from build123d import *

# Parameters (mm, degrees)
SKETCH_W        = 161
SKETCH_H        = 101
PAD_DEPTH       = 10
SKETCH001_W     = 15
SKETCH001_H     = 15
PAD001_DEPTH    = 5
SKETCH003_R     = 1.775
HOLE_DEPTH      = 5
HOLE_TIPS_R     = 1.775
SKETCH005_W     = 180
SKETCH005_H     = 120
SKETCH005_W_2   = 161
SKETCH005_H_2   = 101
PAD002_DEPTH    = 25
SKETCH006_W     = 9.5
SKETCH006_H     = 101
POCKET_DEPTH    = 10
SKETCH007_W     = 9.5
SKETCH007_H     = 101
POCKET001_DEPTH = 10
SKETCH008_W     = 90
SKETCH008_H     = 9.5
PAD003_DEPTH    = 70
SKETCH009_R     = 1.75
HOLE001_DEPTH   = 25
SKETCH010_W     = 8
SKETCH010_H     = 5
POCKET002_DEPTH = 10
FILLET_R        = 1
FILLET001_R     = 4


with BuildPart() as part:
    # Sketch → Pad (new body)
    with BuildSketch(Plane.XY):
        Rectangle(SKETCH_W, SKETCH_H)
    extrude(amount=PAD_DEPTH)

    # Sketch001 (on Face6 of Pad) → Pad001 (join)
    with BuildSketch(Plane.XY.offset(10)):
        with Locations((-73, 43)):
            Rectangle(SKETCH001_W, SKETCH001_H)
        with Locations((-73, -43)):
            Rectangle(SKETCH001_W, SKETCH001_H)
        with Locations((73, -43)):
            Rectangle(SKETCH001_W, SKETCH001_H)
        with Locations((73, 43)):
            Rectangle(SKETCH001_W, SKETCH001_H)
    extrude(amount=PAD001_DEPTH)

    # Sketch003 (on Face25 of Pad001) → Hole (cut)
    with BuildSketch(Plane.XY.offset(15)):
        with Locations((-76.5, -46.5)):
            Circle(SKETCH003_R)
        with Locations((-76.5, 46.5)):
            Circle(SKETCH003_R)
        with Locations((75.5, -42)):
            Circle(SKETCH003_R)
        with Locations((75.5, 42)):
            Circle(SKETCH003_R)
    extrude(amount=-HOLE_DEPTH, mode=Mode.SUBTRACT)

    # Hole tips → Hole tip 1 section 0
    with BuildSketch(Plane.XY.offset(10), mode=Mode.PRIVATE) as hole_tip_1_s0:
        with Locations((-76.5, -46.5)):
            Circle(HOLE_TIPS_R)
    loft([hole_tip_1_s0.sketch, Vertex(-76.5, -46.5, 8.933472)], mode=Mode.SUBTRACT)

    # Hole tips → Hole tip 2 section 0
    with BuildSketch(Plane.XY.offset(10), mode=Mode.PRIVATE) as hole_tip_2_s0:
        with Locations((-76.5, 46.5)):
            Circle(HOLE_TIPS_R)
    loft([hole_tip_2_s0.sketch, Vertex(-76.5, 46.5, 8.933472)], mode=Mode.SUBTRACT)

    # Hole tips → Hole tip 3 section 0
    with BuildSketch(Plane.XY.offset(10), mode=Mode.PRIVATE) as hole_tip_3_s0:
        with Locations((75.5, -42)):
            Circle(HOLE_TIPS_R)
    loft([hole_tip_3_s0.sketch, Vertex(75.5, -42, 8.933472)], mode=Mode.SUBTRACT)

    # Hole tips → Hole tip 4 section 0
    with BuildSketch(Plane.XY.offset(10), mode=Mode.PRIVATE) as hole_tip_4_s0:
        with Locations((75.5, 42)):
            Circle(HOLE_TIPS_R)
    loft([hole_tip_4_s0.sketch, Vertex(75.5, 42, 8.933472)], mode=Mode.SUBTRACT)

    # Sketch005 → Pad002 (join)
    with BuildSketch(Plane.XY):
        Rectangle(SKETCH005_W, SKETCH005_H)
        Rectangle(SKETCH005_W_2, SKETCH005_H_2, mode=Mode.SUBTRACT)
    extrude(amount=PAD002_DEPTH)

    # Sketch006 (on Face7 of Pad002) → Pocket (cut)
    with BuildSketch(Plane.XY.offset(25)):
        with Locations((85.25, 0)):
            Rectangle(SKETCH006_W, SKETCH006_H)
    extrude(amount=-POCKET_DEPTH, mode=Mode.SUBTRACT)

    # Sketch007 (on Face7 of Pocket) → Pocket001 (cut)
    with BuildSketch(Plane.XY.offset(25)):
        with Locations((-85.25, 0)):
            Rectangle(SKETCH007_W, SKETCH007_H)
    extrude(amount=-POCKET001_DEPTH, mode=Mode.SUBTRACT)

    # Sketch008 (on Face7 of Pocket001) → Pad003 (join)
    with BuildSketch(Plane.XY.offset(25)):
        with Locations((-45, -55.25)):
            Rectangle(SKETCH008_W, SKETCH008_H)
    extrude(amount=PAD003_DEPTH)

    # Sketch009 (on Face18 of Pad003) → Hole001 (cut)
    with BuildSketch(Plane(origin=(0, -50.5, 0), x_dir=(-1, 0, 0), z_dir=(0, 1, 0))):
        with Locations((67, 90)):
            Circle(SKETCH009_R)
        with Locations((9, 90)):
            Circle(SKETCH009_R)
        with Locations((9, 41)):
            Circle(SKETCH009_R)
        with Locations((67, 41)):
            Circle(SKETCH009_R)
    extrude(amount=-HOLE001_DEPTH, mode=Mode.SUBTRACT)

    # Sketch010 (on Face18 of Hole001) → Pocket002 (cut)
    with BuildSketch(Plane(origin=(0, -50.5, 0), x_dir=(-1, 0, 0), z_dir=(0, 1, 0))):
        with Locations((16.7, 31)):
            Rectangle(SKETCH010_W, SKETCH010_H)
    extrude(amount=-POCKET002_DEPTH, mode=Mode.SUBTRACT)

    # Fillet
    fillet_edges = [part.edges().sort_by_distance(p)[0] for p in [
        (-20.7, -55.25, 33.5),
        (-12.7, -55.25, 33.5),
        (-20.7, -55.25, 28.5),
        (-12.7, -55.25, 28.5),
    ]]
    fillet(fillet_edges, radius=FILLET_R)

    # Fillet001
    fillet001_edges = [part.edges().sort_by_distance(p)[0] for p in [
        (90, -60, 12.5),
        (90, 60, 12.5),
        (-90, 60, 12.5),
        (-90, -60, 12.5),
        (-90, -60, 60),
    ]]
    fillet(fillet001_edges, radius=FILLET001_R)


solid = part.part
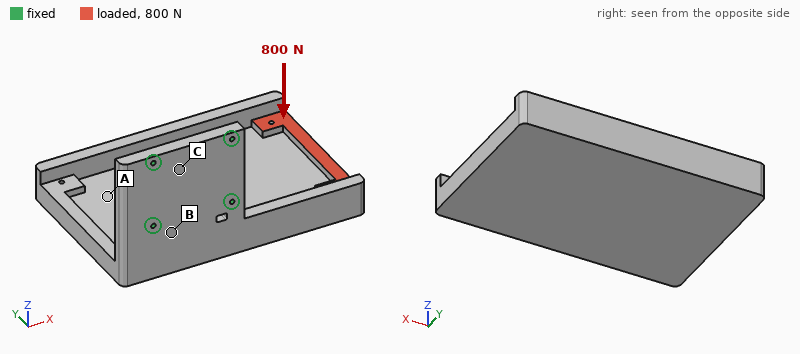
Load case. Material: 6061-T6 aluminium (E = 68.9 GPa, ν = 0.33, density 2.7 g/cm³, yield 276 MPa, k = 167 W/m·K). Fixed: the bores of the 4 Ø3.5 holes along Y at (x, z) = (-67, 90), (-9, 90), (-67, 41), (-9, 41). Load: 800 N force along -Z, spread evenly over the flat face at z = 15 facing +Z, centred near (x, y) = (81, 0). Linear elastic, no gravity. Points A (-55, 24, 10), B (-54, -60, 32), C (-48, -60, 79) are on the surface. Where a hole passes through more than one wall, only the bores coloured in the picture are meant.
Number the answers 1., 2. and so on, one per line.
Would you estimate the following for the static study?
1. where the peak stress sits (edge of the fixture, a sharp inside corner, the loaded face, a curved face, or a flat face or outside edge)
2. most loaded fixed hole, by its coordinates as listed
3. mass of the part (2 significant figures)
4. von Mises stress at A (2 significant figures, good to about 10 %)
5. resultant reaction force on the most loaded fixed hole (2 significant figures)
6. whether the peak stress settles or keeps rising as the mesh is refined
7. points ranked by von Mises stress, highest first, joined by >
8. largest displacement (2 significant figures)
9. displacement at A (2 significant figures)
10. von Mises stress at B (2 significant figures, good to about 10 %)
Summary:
1. edge of the fixture
2. (-9, 41)
3. 920 g
4. 12 MPa
5. 1.7 kN
6. keeps rising
7. B > A > C
8. 1.0 mm
9. 0.35 mm
10. 28 MPa
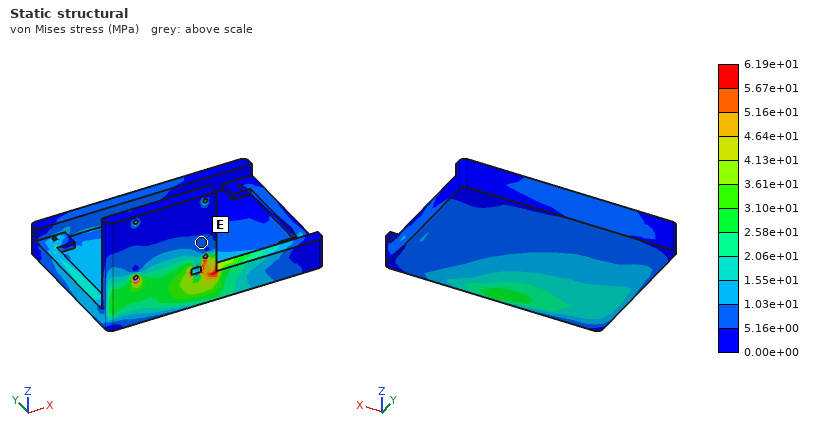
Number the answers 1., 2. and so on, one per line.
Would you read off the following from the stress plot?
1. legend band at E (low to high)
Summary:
1. 5.16e+00 to 1.03e+01 MPa
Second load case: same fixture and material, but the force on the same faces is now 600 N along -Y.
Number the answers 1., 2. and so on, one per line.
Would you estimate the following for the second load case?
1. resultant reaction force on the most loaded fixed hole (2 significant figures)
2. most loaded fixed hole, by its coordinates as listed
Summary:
1. 1.5 kN
2. (-9, 41)
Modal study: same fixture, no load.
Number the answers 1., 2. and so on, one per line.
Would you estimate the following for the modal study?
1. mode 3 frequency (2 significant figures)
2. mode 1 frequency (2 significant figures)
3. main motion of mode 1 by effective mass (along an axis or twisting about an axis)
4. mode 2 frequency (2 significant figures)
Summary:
1. 720 Hz
2. 240 Hz
3. along Z
4. 440 Hz
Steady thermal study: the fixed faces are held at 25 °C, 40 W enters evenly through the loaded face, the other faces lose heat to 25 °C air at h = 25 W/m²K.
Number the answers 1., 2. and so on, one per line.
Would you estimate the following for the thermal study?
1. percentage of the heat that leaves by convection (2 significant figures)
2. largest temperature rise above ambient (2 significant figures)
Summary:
1. 49 %
2. 24 K
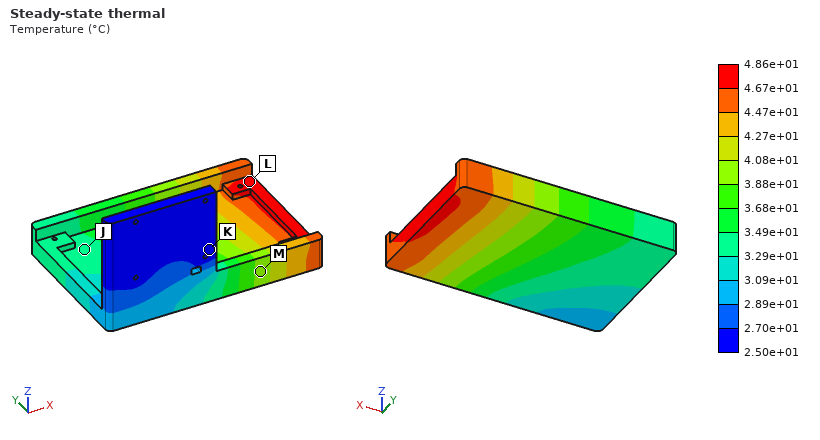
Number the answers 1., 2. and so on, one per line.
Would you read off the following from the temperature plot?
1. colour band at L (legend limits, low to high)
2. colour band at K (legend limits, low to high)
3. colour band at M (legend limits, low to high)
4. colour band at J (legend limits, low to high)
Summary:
1. 4.67e+01 to 4.86e+01 °C
2. 2.50e+01 to 2.70e+01 °C
3. 3.88e+01 to 4.08e+01 °C
4. 3.29e+01 to 3.49e+01 °C
